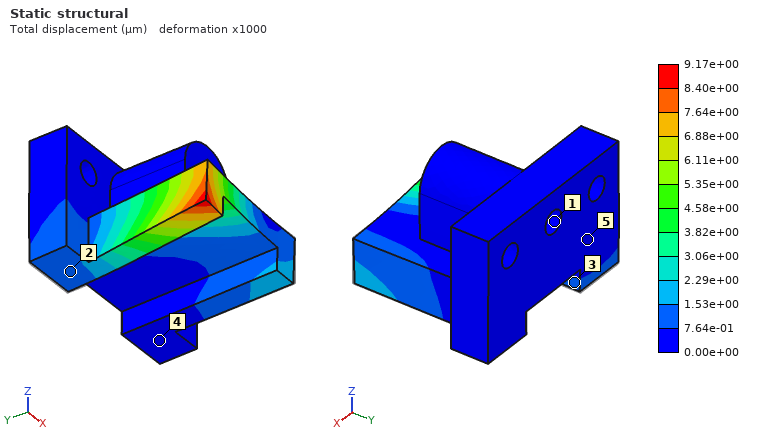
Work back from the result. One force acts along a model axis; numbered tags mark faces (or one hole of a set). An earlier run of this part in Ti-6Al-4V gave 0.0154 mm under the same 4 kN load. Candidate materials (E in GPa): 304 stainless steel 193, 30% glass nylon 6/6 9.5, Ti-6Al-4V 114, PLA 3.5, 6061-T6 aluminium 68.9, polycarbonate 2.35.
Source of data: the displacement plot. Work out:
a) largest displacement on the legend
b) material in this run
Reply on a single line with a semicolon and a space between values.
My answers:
9.17e+00 µm; 304 stainless steel
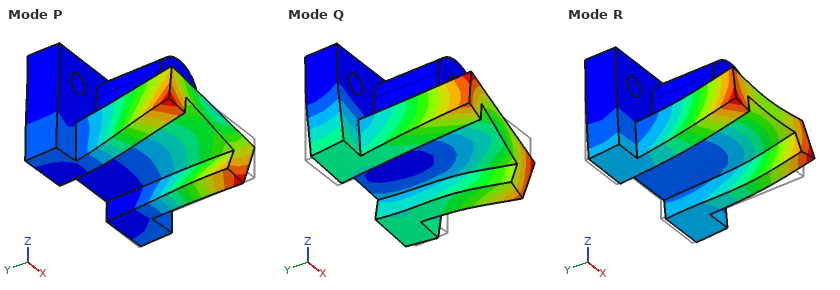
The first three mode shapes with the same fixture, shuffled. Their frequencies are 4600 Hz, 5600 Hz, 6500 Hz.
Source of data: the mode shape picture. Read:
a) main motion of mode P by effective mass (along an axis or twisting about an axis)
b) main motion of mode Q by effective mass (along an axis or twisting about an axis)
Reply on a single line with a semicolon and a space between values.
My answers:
along X; twisting about Z
